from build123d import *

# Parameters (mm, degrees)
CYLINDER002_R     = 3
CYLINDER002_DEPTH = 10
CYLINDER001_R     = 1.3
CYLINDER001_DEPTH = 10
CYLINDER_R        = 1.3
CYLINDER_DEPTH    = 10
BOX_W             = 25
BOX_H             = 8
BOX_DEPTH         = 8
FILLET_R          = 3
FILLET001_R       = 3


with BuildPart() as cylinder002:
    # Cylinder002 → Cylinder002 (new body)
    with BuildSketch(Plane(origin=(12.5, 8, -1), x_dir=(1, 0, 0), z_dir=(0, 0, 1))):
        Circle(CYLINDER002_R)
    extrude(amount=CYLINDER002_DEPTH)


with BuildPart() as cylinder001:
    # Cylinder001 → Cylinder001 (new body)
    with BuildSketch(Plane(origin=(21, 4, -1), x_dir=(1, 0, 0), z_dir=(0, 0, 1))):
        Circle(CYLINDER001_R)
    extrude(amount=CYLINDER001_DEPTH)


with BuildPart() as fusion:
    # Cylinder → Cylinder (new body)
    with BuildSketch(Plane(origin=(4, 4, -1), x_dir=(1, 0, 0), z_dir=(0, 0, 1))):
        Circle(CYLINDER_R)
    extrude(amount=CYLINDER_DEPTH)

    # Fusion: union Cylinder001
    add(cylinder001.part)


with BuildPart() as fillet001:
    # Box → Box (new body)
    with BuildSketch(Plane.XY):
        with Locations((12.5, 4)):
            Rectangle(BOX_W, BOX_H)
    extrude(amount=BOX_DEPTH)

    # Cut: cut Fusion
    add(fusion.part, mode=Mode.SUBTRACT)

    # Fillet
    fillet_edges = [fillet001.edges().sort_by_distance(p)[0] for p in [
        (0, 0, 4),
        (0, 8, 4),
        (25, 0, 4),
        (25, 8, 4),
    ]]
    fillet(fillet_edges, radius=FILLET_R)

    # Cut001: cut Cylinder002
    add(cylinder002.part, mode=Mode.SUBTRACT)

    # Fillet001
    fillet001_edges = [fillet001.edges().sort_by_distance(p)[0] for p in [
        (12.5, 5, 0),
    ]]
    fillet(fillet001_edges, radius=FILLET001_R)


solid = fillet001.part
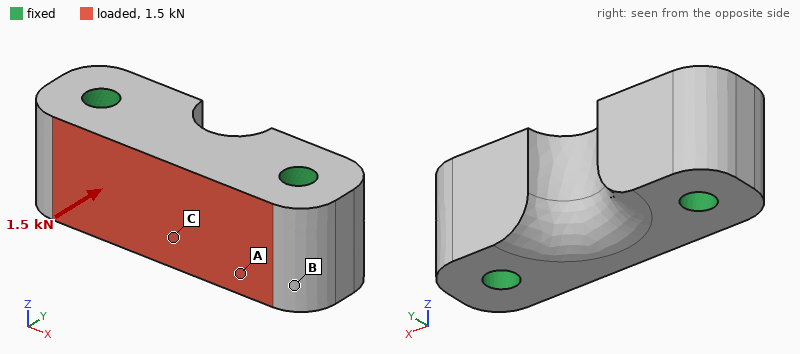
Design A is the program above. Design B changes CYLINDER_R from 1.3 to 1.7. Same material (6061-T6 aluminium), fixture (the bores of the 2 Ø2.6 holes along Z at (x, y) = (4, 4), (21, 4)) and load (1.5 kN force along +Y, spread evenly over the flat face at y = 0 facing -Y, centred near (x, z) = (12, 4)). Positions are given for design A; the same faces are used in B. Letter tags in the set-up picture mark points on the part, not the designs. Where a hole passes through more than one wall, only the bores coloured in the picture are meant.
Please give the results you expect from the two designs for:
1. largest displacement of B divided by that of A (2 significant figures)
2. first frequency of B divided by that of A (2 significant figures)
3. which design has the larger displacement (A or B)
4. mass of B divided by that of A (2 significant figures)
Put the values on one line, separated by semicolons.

0.89; 1.1; A; 0.98
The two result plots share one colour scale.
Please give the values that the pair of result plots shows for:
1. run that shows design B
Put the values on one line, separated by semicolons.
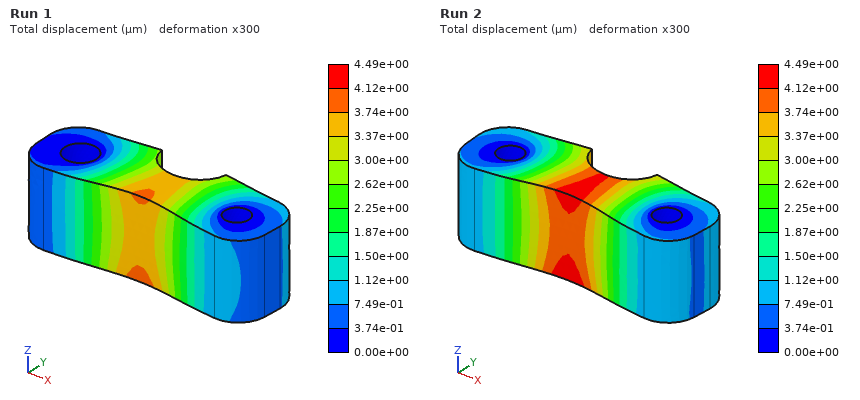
Run 1
